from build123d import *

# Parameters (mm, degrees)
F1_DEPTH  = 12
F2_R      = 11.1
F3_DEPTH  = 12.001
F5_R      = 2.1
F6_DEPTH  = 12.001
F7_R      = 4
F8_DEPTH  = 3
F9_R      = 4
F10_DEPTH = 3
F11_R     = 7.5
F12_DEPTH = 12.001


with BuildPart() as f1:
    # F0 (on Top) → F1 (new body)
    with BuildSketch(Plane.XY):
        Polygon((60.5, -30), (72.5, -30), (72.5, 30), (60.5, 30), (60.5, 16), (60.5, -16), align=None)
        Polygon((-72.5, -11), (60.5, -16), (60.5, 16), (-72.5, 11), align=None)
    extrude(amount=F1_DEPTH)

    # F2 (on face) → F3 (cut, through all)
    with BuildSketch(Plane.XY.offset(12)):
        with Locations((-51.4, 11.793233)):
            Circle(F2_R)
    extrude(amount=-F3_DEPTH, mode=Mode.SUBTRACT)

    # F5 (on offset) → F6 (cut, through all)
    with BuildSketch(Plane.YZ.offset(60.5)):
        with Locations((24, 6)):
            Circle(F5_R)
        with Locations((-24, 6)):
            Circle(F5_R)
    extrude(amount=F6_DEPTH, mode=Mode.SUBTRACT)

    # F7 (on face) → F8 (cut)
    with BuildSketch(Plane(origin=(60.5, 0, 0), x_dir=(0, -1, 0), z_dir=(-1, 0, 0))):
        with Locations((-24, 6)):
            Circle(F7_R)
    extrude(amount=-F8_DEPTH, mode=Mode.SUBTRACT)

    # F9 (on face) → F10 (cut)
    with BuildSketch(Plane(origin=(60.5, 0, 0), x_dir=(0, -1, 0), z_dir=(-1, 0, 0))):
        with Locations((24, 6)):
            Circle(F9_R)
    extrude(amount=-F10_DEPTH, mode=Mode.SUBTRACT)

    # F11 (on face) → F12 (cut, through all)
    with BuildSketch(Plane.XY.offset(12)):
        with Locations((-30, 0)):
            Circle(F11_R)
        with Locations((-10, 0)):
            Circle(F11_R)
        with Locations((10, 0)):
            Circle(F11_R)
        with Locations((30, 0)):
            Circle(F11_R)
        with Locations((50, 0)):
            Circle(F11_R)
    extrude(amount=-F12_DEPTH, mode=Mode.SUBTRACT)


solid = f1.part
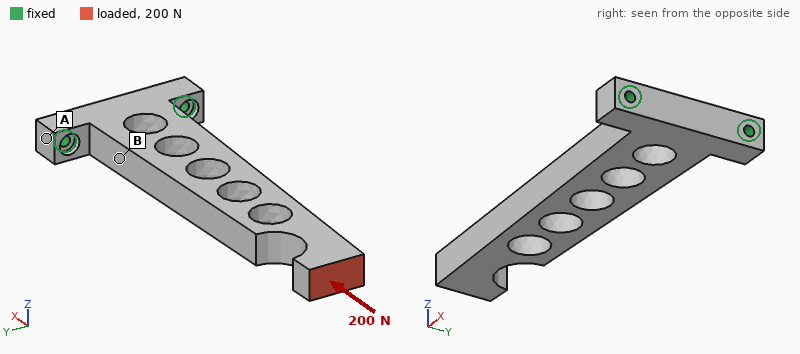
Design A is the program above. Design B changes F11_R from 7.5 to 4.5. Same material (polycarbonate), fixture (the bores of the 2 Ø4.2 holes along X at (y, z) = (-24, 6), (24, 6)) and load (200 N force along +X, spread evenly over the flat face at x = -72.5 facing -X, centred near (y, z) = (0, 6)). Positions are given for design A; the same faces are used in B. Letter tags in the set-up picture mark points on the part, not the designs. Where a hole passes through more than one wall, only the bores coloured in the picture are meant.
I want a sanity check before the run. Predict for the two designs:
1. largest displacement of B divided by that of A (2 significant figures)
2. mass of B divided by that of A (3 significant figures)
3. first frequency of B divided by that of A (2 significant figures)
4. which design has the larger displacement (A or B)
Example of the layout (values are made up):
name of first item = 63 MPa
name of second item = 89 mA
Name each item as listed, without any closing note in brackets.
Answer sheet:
largest displacement of B divided by that of A = 0.80
mass of B divided by that of A = 1.18
first frequency of B divided by that of A = 1.0
which design has the larger displacement = A
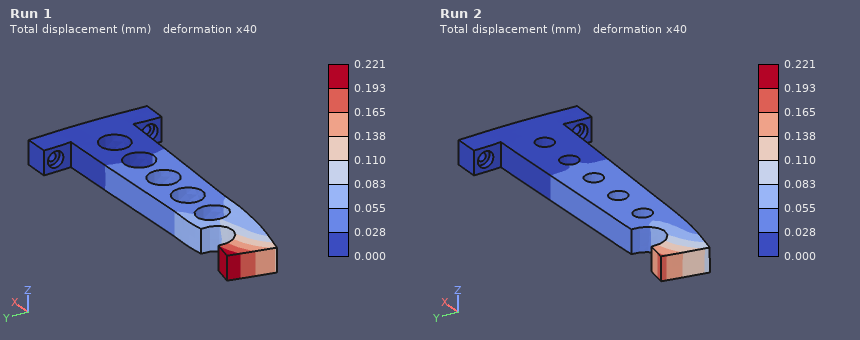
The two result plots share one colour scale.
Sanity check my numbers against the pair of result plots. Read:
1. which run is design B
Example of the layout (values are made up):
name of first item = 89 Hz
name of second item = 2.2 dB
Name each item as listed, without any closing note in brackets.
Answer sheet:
which run is design B = Run 2
